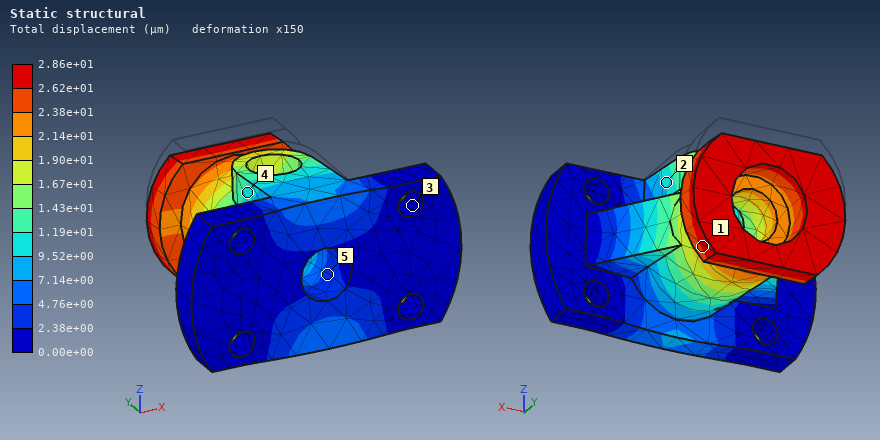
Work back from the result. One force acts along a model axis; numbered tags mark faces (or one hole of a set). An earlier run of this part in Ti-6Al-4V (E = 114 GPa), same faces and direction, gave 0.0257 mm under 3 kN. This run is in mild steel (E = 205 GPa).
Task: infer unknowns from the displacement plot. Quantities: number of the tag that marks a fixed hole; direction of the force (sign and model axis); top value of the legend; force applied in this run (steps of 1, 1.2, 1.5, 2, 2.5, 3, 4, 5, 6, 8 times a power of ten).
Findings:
3
-Z
2.86e+01 µm
6 kN
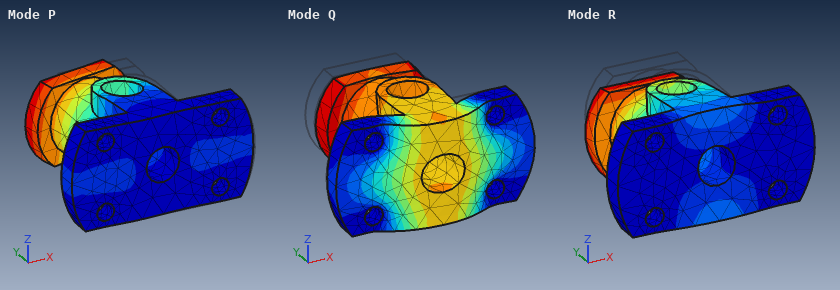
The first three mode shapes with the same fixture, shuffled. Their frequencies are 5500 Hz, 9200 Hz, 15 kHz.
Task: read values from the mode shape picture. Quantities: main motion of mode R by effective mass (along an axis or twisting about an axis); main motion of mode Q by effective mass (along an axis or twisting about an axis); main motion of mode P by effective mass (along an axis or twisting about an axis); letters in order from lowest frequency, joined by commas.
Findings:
along Z
along Y
along X
R, P, Q
